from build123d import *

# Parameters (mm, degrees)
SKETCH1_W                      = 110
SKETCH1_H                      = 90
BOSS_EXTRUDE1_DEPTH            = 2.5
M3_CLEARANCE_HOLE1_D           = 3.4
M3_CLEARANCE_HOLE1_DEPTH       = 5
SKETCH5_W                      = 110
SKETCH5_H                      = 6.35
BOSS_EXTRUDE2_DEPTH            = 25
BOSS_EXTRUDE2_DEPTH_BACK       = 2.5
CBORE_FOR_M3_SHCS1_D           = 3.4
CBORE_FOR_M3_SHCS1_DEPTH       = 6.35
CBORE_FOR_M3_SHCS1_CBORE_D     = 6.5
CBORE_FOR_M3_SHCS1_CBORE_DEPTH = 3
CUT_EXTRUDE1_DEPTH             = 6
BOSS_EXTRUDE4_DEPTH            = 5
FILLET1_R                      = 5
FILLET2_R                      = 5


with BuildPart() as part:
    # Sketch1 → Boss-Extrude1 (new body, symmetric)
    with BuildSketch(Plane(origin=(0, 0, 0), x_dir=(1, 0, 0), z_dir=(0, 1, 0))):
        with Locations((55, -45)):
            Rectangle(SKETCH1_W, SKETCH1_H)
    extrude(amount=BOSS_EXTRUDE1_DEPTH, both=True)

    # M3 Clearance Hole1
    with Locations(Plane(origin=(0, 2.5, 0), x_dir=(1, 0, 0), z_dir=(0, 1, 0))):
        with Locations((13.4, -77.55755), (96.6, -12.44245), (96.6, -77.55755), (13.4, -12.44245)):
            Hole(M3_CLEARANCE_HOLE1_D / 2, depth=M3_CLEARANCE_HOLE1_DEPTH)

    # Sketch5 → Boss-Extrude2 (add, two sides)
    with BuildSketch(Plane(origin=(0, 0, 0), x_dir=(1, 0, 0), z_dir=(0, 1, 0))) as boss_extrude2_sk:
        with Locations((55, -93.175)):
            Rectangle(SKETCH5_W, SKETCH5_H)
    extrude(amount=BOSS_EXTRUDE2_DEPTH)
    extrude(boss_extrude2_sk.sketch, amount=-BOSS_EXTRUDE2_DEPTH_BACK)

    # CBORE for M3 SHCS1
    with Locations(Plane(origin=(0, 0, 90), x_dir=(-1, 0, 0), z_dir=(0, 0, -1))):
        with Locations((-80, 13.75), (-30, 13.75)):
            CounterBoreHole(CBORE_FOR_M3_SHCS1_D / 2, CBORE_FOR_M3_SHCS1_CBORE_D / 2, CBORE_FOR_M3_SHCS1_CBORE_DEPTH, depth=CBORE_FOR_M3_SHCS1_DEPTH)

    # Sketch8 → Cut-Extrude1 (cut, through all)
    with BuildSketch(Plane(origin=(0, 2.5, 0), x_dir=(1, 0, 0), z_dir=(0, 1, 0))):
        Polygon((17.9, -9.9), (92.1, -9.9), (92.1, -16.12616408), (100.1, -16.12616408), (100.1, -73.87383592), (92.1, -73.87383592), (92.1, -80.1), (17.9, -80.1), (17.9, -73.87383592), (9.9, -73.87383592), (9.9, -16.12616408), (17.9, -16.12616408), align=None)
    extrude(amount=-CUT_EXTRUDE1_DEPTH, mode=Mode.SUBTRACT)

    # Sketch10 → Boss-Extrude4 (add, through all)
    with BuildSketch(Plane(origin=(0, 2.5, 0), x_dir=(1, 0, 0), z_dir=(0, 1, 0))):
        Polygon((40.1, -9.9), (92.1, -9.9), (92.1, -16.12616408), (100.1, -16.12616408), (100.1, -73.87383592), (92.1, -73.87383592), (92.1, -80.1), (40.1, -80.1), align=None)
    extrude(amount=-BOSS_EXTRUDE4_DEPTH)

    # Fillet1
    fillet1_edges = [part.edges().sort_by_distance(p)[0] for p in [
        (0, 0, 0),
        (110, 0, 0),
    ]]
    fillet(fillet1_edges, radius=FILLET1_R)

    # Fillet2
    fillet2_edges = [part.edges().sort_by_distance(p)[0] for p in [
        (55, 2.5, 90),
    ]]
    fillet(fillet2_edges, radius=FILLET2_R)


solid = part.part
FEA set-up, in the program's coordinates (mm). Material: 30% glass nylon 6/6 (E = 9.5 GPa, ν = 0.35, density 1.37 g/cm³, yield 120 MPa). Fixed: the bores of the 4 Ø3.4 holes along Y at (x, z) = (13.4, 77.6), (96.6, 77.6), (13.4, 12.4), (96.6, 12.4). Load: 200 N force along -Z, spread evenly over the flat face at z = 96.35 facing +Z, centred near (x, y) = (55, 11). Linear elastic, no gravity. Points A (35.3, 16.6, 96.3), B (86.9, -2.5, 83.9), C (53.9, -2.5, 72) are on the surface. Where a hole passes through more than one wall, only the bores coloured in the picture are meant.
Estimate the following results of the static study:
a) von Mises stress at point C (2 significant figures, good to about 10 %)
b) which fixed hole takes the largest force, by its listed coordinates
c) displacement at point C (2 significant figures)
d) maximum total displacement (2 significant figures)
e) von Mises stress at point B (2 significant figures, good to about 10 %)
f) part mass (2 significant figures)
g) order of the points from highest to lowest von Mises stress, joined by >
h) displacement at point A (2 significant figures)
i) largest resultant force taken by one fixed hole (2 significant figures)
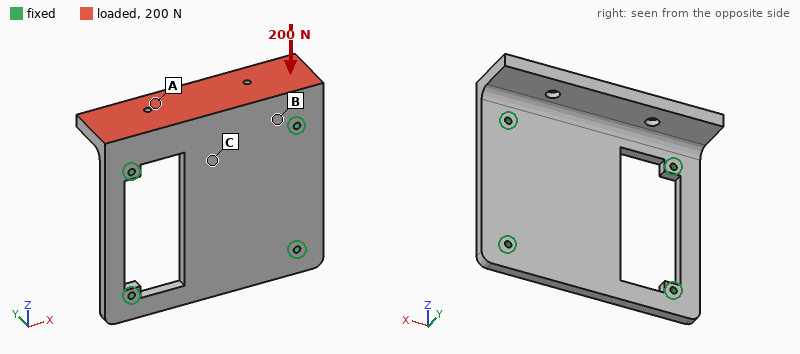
2.6 MPa
(96.6, 77.6)
0.022 mm
0.14 mm
4.7 MPa
80 g
B > C > A
0.11 mm
88 N
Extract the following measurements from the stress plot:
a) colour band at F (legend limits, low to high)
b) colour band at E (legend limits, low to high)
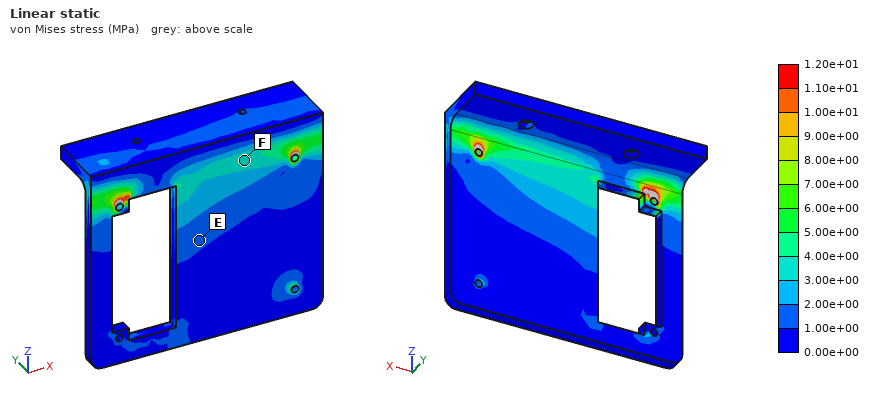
3.00e+00 to 4.00e+00 MPa
1.00e+00 to 2.00e+00 MPa
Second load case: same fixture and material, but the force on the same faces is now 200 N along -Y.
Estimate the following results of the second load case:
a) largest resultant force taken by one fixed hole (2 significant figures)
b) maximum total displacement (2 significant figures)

120 N
0.18 mm
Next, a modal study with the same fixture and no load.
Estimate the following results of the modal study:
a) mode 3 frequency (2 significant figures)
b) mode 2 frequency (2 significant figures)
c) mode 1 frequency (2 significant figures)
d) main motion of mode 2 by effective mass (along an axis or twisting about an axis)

2100 Hz
1400 Hz
1100 Hz
along Y
